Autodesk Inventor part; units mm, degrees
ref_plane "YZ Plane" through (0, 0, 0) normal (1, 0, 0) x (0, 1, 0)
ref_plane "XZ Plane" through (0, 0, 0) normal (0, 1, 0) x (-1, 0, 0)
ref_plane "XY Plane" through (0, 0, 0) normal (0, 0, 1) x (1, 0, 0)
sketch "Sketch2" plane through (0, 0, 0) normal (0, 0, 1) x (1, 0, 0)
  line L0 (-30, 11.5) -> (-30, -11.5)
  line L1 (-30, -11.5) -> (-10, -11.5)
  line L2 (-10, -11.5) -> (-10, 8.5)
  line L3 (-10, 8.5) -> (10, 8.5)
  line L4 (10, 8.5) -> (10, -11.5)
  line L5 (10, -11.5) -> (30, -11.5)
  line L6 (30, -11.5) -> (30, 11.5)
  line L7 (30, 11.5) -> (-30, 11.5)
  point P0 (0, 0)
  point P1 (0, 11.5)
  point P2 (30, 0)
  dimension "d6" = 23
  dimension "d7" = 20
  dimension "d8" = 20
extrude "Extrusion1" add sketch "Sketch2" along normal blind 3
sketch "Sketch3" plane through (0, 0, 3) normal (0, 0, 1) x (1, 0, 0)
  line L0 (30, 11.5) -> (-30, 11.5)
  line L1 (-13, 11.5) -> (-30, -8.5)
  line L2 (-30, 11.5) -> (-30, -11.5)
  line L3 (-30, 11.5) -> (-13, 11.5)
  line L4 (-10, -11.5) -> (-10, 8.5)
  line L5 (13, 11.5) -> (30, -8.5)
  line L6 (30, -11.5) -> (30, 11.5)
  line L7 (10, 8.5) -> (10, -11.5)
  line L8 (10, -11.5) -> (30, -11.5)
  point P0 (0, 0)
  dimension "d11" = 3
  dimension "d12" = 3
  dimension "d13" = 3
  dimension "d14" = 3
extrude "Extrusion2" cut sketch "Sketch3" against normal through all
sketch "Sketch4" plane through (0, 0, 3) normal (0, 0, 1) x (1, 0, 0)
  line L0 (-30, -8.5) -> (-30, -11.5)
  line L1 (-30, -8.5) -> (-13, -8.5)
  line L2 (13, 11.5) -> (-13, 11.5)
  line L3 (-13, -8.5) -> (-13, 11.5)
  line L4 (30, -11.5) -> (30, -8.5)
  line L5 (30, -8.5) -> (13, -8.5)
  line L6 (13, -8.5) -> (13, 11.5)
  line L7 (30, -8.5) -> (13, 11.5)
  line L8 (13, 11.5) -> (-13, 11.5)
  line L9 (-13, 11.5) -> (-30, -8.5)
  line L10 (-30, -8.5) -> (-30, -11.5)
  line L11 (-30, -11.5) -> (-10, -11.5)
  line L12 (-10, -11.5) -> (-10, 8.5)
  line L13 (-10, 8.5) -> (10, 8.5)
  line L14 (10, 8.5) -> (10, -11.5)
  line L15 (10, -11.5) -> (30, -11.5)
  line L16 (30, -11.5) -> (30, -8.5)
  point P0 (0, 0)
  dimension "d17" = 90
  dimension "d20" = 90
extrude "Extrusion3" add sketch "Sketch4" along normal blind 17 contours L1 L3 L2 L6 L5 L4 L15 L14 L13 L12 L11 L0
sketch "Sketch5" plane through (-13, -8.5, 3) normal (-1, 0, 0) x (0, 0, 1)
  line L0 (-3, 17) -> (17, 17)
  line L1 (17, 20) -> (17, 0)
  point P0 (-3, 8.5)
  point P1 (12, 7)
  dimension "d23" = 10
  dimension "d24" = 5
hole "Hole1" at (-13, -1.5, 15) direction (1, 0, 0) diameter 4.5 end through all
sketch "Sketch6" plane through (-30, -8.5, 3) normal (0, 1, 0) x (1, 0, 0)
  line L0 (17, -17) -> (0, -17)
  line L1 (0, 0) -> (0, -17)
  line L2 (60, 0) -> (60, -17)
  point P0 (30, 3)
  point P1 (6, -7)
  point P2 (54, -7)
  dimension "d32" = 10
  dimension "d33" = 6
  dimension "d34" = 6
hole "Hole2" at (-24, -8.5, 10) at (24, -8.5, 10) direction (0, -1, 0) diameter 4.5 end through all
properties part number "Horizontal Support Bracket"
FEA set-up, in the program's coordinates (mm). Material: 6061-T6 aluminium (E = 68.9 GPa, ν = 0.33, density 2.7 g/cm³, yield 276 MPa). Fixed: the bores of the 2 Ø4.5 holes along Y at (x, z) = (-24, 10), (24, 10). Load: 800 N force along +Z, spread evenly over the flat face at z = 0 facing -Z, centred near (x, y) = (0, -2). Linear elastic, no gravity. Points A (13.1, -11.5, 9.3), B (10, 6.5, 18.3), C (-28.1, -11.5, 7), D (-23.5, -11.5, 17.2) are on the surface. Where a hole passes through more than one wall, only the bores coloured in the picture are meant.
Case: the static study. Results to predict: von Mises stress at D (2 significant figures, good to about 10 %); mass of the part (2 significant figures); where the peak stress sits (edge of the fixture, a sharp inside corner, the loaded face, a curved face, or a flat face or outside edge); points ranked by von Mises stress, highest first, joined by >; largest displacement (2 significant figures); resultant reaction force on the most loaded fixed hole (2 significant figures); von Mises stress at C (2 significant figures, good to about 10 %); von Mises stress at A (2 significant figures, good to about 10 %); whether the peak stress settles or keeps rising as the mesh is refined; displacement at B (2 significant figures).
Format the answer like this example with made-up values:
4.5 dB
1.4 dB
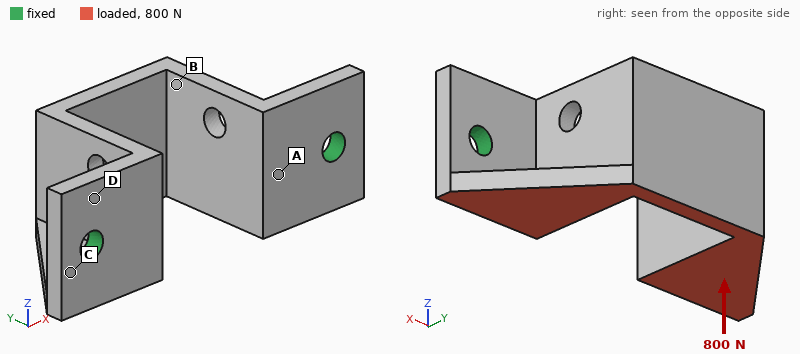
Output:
49 MPa
18 g
edge of the fixture
C > D > A > B
0.12 mm
400 N
66 MPa
31 MPa
keeps rising
0.098 mm
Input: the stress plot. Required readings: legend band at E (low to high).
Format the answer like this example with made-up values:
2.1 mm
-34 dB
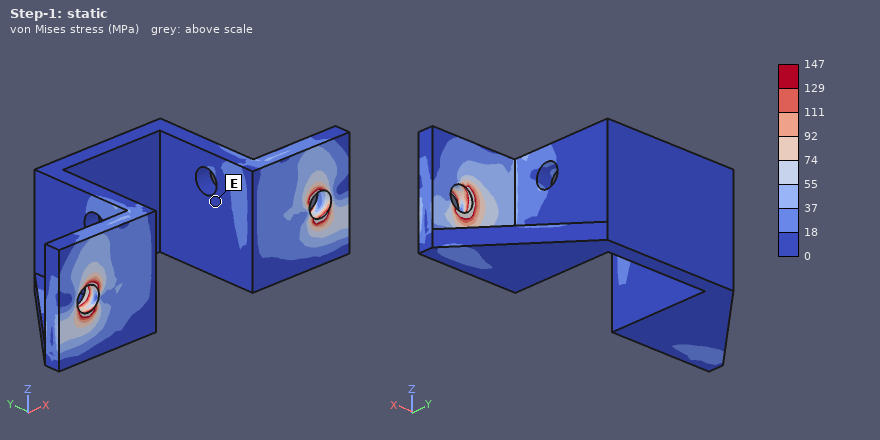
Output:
0 to 18 MPa
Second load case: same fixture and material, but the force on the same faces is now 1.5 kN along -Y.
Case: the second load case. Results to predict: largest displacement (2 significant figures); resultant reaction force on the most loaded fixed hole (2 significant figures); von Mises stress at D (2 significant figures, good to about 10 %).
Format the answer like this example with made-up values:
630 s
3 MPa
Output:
0.16 mm
790 N
47 MPa
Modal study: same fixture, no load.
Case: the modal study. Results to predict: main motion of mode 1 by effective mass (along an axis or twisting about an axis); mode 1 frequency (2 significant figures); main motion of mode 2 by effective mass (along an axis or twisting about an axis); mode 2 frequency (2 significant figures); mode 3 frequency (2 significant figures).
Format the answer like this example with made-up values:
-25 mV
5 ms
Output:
along Z
3300 Hz
along X
5500 Hz
6800 Hz
